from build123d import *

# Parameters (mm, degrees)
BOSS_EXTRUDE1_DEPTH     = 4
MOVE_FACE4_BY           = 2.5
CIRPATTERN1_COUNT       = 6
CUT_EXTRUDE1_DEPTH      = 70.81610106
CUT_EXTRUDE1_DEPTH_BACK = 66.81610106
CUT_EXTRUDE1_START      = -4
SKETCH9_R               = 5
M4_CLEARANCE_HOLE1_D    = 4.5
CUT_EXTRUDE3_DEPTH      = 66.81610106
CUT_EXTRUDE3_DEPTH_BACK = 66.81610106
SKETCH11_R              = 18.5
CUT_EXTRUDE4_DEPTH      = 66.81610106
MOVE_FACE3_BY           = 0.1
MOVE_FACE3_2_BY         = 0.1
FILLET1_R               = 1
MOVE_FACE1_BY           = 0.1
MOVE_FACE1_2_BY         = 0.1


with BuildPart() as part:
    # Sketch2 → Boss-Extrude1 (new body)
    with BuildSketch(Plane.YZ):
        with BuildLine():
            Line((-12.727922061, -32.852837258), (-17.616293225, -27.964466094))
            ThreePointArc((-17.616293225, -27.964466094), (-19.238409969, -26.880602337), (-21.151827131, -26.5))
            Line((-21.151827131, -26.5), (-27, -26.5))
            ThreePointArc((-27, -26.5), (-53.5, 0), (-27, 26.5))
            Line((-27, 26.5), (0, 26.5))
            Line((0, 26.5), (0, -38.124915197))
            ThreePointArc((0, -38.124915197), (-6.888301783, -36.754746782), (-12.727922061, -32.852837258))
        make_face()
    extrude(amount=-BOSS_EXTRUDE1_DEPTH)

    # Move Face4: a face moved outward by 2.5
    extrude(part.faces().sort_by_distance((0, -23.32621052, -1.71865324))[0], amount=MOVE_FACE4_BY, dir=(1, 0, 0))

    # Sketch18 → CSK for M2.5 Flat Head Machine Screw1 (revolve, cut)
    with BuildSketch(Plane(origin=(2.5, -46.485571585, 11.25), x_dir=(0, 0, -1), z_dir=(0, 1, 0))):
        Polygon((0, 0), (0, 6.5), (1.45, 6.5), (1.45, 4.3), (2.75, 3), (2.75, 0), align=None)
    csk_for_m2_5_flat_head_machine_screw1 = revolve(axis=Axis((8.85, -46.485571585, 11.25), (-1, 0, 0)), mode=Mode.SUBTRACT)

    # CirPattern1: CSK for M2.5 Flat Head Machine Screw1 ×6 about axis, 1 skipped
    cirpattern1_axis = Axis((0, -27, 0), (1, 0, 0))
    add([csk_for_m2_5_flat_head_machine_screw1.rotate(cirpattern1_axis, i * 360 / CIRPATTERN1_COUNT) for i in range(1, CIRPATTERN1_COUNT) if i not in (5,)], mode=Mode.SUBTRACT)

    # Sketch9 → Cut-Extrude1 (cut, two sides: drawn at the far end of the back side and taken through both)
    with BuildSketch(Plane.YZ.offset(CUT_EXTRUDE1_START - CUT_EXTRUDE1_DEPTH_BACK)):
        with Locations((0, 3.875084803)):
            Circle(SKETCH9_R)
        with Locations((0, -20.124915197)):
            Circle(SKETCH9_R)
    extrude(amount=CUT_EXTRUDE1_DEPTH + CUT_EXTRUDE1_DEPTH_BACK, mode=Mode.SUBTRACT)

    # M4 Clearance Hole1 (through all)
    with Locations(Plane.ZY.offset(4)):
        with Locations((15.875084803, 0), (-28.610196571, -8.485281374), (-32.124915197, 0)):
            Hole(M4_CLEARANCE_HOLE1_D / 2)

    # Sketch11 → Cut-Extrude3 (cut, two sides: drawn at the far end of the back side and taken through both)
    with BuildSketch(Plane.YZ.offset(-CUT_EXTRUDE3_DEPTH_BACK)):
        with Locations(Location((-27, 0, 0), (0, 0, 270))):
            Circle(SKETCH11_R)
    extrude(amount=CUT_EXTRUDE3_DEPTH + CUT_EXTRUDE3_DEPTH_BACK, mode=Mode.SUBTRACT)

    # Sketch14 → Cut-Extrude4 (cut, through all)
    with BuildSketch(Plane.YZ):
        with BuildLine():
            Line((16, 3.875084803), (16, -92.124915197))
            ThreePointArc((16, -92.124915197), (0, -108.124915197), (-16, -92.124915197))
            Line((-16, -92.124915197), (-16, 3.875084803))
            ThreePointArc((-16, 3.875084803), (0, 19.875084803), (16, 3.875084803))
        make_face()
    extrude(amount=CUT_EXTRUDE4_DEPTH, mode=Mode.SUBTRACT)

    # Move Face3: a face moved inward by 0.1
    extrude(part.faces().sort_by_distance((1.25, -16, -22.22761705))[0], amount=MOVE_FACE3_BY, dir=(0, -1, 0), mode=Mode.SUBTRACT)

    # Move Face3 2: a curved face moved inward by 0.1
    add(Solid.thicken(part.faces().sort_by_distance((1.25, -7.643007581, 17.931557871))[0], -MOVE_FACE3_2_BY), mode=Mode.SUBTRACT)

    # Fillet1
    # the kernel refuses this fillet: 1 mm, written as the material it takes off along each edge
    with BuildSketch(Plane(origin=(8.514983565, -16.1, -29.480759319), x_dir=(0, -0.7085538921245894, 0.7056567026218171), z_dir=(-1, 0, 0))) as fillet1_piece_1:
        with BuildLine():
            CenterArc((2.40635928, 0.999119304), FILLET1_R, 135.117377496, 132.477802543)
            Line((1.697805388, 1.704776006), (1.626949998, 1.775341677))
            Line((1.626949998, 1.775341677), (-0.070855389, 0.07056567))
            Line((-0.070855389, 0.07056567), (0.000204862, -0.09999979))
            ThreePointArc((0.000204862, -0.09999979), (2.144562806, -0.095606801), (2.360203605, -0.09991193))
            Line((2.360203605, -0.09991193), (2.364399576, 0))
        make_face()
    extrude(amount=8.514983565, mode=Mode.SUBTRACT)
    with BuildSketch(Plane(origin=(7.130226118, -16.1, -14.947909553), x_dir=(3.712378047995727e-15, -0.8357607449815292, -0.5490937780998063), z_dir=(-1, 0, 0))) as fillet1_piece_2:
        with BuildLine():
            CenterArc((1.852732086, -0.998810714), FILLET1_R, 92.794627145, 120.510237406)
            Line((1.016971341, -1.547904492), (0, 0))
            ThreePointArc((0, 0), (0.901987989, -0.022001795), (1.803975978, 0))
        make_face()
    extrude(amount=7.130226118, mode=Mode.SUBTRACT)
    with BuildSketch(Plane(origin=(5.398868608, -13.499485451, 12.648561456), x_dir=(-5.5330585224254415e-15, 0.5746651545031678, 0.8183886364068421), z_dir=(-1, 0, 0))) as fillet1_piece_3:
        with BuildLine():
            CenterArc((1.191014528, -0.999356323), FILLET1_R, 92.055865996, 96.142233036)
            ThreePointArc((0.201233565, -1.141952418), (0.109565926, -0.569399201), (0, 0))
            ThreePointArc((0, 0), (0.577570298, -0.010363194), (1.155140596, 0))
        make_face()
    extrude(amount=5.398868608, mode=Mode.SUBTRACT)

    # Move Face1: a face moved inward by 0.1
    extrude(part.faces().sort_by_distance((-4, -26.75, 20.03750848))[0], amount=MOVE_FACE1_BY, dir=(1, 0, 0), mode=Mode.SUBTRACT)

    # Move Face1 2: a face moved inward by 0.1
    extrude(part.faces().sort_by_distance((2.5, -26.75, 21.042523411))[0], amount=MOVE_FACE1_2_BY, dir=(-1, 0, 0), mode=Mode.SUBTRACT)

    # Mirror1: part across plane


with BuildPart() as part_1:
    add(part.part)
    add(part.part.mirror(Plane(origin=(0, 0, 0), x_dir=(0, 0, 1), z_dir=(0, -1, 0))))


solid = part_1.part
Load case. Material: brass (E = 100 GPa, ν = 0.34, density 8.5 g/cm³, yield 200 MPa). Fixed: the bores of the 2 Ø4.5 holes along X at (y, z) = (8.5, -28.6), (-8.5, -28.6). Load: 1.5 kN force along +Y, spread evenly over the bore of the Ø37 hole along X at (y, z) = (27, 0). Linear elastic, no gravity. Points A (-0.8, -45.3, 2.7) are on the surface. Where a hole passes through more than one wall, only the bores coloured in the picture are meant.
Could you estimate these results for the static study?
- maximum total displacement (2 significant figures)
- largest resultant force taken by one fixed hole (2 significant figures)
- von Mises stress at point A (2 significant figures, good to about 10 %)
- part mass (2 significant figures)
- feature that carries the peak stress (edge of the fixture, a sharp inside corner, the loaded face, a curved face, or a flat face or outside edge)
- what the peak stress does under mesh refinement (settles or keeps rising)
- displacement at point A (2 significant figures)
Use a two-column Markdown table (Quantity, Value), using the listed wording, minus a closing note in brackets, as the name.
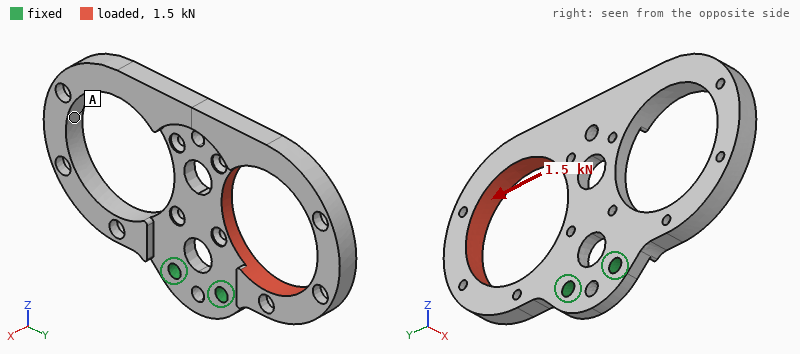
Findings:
| Quantity | Value |
|---|---|
| maximum total displacement | 0.15 mm |
| largest resultant force taken by one fixed hole | 2.0 kN |
| von Mises stress at point A | 21 MPa |
| part mass | 130 g |
| feature that carries the peak stress | edge of the fixture |
| what the peak stress does under mesh refinement | keeps rising |
| displacement at point A | 0.11 mm |
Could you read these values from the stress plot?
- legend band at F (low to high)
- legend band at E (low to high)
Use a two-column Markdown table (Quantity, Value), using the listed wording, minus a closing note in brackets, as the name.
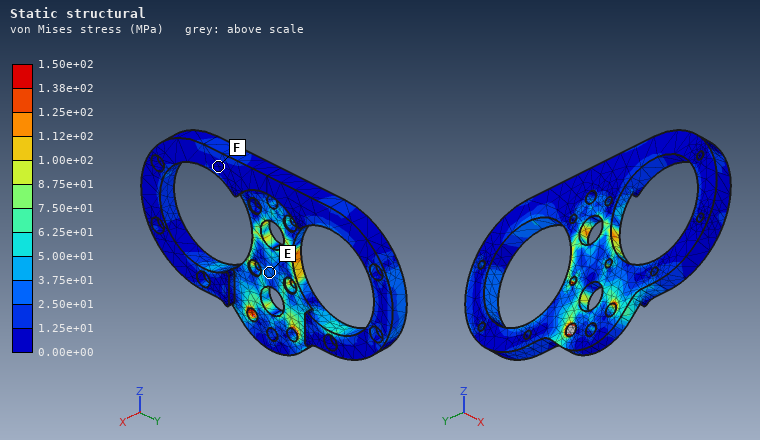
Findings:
| Quantity | Value |
|---|---|
| legend band at F | 0.00e+00 to 1.25e+01 MPa |
| legend band at E | 2.50e+01 to 3.75e+01 MPa |
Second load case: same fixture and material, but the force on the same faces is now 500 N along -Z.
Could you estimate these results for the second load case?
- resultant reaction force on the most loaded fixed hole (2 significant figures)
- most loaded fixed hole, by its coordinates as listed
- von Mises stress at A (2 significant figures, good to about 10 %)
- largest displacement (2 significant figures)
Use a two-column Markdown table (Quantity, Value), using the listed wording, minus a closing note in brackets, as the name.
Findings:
| Quantity | Value |
|---|---|
| resultant reaction force on the most loaded fixed hole | 870 N |
| most loaded fixed hole, by its coordinates as listed | (8.5, -28.6) |
| von Mises stress at A | 6.7 MPa |
| largest displacement | 61 µm |
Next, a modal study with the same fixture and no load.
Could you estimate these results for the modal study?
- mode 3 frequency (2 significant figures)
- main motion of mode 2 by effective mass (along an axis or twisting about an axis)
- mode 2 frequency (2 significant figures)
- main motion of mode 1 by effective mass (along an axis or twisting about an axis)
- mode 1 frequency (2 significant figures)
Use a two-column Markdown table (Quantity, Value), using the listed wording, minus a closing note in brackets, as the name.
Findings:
| Quantity | Value |
|---|---|
| mode 3 frequency | 1300 Hz |
| main motion of mode 2 by effective mass | twisting about Z |
| mode 2 frequency | 600 Hz |
| main motion of mode 1 by effective mass | along X |
| mode 1 frequency | 430 Hz |
